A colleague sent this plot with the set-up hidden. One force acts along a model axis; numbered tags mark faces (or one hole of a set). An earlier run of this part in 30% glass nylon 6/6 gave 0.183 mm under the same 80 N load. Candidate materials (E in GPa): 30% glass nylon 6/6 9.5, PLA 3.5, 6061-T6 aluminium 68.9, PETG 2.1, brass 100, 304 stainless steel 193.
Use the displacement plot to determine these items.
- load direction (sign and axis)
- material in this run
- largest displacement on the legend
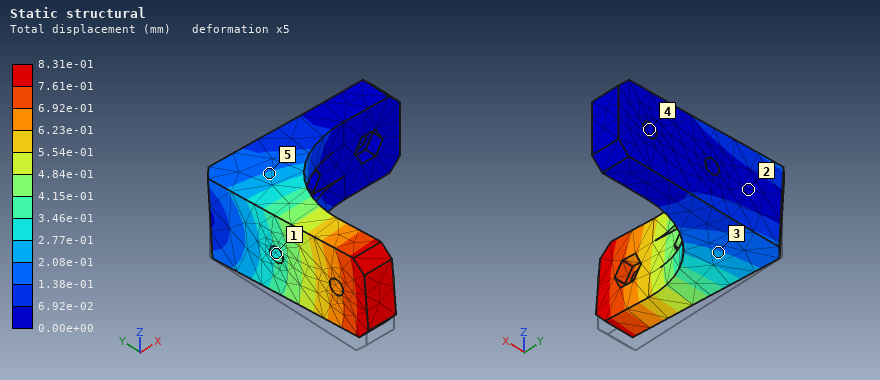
+Z
PETG
8.31e-01 mm
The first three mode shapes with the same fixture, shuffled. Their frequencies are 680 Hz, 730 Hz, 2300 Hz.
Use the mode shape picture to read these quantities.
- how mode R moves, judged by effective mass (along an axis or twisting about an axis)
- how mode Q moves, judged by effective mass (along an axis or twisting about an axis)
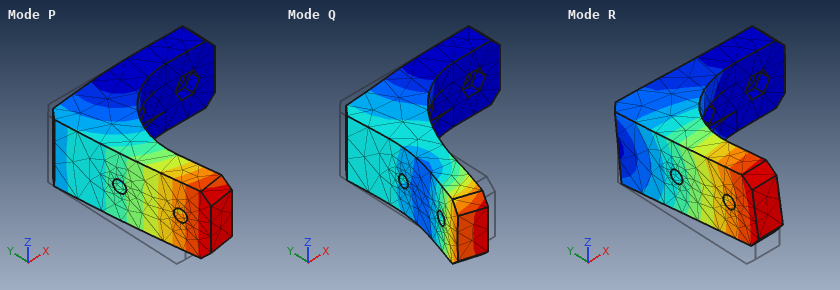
along Z
along Y
